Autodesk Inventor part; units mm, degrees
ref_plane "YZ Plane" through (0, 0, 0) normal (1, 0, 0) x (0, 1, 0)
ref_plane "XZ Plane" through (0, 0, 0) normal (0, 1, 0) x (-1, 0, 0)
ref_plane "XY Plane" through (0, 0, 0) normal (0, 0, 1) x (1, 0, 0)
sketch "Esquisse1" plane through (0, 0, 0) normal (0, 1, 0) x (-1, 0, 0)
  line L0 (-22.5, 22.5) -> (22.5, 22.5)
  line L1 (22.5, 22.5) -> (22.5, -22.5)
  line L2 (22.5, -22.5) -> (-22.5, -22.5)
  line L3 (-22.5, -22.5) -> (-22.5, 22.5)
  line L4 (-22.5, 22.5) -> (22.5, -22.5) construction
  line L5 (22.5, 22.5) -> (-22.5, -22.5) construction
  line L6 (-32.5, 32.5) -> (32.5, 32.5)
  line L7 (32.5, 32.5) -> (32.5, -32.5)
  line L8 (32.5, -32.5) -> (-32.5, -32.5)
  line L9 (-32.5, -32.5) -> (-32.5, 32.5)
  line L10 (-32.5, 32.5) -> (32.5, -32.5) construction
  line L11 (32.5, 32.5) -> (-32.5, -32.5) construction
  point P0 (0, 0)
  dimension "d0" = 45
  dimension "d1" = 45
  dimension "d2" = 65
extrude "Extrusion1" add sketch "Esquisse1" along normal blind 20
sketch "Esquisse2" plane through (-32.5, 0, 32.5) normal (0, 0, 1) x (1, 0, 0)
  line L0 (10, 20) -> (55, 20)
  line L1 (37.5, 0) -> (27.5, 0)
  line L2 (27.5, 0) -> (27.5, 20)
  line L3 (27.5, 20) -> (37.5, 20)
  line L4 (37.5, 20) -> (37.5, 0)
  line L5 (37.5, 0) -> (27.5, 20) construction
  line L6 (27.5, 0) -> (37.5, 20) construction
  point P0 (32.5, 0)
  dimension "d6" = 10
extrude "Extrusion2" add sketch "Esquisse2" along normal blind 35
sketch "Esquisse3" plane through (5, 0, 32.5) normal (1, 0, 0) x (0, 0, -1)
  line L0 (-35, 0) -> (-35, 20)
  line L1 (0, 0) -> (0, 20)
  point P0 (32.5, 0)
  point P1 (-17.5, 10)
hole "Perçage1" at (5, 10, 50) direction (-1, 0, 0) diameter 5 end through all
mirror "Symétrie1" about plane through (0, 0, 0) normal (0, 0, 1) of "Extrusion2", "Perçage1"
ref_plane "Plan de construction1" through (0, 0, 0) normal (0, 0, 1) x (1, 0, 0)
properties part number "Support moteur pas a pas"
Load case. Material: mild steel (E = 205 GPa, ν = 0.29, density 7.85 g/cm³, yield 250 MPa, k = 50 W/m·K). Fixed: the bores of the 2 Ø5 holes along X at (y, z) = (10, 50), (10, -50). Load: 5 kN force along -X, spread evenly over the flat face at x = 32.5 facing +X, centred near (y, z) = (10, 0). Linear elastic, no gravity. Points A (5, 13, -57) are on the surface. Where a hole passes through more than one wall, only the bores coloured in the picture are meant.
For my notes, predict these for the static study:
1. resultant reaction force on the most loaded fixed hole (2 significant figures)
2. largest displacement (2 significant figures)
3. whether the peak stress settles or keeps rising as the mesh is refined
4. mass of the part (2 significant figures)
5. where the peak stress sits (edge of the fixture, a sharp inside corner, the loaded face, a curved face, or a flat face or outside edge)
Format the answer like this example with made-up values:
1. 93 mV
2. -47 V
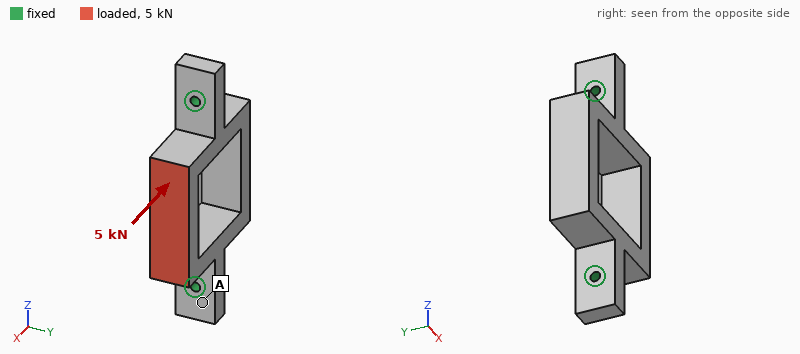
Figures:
1. 2.6 kN
2. 19 µm
3. keeps rising
4. 450 g
5. edge of the fixture
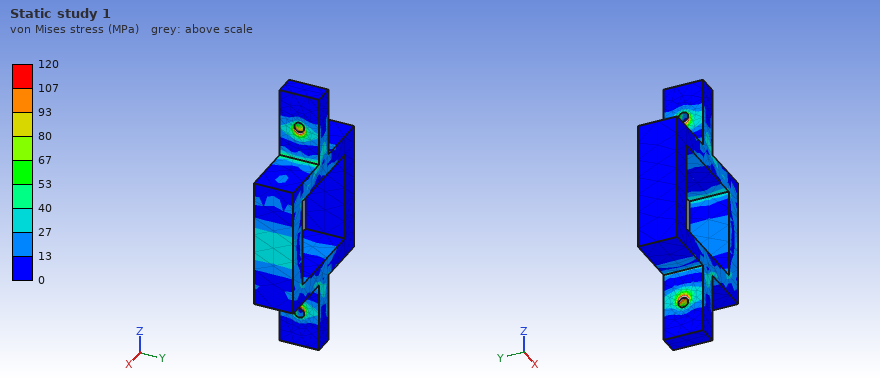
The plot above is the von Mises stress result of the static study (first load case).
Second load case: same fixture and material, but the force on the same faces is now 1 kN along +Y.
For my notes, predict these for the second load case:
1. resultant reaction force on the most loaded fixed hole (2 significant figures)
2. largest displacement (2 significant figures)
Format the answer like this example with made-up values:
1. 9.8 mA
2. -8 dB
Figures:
1. 500 N
2. 37 µm
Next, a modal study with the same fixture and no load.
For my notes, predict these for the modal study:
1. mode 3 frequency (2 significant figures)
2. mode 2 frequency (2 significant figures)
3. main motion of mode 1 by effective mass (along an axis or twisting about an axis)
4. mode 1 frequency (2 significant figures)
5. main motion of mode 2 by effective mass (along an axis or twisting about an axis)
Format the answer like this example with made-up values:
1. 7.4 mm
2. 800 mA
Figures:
1. 5200 Hz
2. 3800 Hz
3. twisting about Z
4. 2300 Hz
5. along Y
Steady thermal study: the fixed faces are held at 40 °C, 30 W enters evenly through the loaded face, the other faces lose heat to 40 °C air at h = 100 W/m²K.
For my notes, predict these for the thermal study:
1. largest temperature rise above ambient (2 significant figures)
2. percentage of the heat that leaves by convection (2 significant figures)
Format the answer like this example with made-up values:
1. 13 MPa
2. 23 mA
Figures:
1. 44 K
2. 66 %
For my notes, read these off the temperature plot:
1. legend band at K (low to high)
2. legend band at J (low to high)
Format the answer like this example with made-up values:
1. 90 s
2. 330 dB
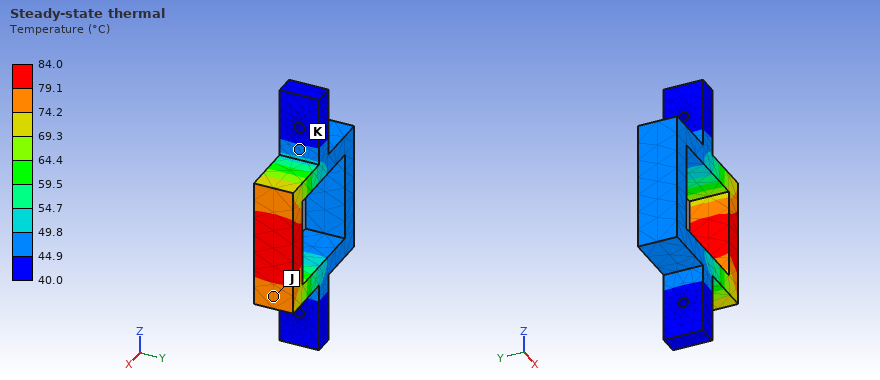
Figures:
1. 44.9 to 49.8 °C
2. 74.2 to 79.1 °C
